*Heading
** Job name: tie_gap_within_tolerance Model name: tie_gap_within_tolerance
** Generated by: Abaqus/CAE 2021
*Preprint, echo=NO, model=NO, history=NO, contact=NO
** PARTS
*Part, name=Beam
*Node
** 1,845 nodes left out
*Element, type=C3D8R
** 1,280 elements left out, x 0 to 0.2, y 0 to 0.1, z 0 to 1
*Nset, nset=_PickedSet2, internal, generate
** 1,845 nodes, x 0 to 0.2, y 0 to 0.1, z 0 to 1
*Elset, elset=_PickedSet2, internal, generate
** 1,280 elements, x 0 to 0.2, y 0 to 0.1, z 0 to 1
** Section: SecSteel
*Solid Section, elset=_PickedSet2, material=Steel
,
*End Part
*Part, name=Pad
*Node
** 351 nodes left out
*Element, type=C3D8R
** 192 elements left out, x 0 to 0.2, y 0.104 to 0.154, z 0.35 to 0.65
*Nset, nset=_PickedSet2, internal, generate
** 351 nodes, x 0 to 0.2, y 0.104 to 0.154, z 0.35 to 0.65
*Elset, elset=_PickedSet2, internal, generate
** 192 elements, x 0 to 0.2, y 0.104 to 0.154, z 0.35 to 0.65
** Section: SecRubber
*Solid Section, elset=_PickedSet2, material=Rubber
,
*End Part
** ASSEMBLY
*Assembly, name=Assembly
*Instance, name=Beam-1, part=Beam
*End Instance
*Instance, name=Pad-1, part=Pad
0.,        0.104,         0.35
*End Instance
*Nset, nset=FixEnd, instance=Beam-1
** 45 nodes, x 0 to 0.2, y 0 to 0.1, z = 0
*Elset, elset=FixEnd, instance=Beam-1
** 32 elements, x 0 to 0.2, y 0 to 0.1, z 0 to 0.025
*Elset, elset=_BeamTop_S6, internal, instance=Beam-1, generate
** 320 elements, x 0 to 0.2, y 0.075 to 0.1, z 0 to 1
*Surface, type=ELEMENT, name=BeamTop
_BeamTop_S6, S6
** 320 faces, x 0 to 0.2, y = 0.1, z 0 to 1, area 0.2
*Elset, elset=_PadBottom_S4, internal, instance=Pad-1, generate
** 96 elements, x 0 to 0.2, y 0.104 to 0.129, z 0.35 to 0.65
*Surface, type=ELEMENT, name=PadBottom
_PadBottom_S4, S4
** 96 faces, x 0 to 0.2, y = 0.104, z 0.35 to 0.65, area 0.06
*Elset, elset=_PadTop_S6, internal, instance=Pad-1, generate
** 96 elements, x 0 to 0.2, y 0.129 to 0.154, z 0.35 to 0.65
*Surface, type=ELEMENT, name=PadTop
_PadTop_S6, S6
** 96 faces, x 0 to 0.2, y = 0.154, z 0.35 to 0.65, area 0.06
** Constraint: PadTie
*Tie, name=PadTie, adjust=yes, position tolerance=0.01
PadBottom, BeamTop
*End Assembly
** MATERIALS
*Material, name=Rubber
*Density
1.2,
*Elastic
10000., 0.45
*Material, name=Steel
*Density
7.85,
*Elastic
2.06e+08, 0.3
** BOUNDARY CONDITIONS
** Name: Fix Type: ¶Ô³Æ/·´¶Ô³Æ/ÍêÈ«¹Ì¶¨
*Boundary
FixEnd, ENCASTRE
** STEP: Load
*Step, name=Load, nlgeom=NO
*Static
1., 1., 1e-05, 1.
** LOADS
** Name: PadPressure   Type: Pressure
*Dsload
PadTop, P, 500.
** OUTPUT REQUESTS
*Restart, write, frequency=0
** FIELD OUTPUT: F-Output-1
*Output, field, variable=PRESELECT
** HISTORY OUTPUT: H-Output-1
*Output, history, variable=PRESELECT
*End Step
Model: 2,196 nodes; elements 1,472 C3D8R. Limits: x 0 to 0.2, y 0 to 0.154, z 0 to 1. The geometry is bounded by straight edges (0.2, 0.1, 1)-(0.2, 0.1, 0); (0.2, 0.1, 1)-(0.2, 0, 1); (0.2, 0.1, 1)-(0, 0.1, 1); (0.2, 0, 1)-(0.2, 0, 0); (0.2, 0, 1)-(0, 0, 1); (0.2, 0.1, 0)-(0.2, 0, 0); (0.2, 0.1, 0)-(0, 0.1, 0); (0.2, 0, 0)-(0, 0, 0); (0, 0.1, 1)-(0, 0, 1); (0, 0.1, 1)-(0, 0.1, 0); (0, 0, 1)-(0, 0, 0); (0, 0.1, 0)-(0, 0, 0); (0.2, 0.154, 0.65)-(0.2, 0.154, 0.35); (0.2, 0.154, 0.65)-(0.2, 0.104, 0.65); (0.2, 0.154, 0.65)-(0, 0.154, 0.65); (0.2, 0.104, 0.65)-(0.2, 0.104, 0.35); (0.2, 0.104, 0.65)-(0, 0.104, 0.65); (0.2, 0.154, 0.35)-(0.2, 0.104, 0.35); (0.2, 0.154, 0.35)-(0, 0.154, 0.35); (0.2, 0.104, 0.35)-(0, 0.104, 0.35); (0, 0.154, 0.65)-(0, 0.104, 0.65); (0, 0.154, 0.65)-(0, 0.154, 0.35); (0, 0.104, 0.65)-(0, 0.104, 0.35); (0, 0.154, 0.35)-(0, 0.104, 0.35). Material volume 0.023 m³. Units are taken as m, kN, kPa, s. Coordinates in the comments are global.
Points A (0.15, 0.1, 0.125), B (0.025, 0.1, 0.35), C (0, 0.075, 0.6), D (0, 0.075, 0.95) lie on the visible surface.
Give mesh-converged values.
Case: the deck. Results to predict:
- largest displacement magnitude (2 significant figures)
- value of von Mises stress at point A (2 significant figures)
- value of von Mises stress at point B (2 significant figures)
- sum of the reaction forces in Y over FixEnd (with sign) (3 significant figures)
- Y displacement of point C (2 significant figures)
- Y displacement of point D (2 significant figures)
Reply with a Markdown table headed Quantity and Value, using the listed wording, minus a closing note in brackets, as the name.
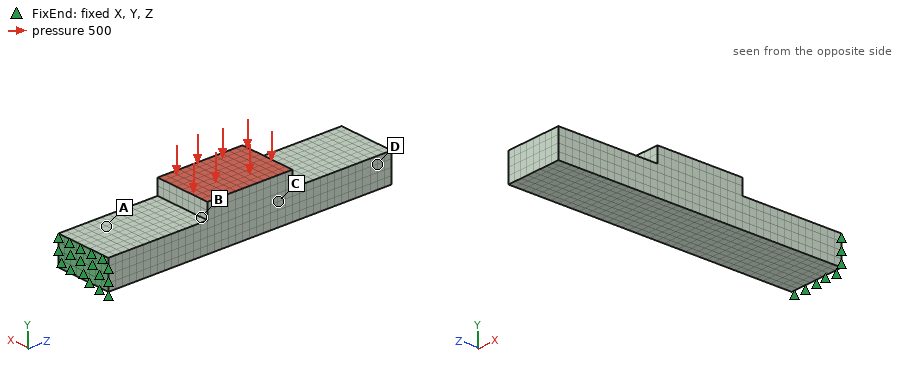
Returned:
| Quantity | Value |
|---|---|
| largest displacement magnitude | 0.0048 m |
| value of von Mises stress at point A | 33000 kPa |
| value of von Mises stress at point B | 14000 kPa |
| sum of the reaction forces in Y over FixEnd (with sign) | 30.0 kN |
| Y displacement of point C | -4.8e-04 m |
| Y displacement of point D | -8.7e-04 m |
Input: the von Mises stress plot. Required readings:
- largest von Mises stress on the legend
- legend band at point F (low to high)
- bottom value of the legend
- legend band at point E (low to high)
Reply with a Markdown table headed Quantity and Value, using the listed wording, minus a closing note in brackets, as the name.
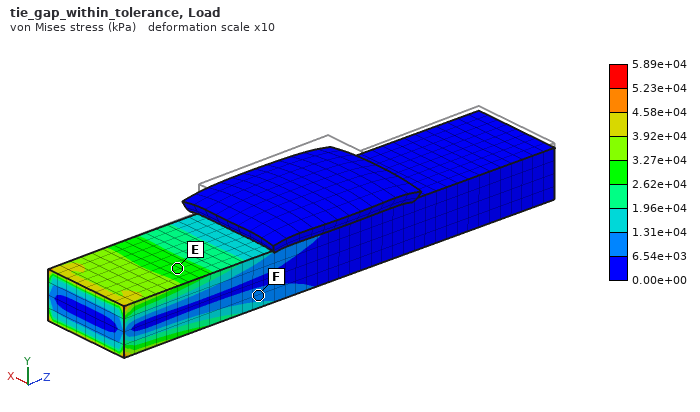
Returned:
| Quantity | Value |
|---|---|
| largest von Mises stress on the legend | 5.89e+04 kPa |
| legend band at point F | 6.54e+03 to 1.31e+04 kPa |
| bottom value of the legend | 0.00e+00 kPa |
| legend band at point E | 2.62e+04 to 3.27e+04 kPa |
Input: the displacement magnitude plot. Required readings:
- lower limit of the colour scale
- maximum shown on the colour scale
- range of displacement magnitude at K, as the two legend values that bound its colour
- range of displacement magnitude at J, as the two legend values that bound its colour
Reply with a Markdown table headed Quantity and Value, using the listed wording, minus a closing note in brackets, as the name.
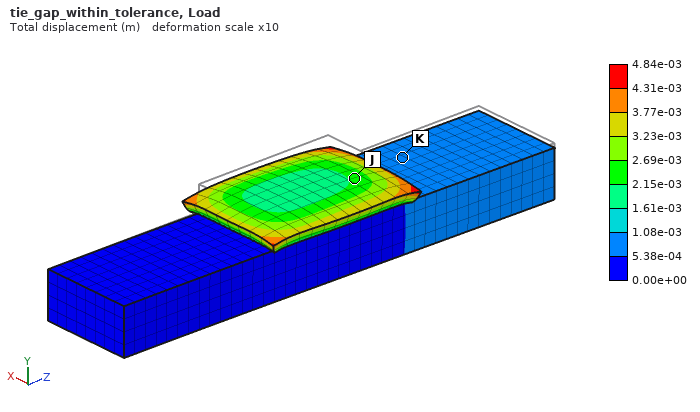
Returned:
| Quantity | Value |
|---|---|
| lower limit of the colour scale | 0.00e+00 m |
| maximum shown on the colour scale | 4.84e-03 m |
| range of displacement magnitude at K, as the two legend values that bound its colour | 5.38e-04 to 1.08e-03 m |
| range of displacement magnitude at J, as the two legend values that bound its colour | 2.15e-03 to 2.69e-03 m |
